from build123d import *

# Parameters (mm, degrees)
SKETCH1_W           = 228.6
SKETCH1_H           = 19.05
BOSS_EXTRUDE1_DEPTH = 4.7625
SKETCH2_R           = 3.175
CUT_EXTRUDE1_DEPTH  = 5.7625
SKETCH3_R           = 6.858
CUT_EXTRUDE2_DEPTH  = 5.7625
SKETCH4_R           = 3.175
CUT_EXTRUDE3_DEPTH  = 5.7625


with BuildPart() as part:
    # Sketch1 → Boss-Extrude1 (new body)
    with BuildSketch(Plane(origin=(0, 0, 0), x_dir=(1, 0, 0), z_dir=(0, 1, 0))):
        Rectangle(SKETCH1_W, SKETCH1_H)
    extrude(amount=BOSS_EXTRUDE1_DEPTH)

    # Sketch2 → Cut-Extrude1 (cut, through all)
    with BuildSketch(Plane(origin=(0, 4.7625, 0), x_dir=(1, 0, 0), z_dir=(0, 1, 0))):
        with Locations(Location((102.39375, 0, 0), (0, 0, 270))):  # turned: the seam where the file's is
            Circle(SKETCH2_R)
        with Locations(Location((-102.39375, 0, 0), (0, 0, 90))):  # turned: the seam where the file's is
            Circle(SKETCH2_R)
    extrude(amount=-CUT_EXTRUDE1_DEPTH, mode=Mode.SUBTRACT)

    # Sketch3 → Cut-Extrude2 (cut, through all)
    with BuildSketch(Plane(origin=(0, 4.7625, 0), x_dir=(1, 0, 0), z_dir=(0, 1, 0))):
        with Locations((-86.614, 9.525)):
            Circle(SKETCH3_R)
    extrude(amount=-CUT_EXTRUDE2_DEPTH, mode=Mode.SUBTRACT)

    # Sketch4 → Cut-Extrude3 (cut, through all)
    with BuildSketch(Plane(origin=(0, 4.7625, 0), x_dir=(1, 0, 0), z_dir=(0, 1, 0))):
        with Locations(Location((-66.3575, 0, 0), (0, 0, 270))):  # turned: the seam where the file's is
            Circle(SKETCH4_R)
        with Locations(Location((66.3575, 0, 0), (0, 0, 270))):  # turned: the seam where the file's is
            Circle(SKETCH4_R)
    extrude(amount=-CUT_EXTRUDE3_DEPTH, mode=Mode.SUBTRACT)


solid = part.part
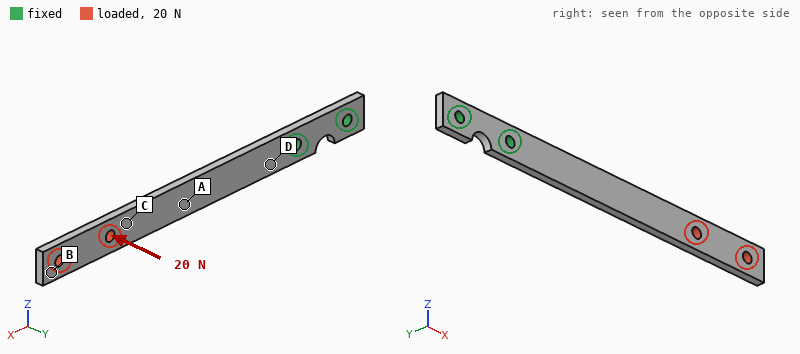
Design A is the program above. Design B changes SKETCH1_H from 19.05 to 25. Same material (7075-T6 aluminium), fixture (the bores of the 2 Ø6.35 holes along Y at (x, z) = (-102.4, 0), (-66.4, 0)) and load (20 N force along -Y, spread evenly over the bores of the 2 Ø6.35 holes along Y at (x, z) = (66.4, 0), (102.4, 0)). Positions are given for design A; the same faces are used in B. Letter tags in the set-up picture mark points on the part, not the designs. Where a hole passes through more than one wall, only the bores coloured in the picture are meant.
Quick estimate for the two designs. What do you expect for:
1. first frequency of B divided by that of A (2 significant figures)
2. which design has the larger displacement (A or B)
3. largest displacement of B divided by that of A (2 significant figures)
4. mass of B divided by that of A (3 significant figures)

0.99
A
0.77
1.32
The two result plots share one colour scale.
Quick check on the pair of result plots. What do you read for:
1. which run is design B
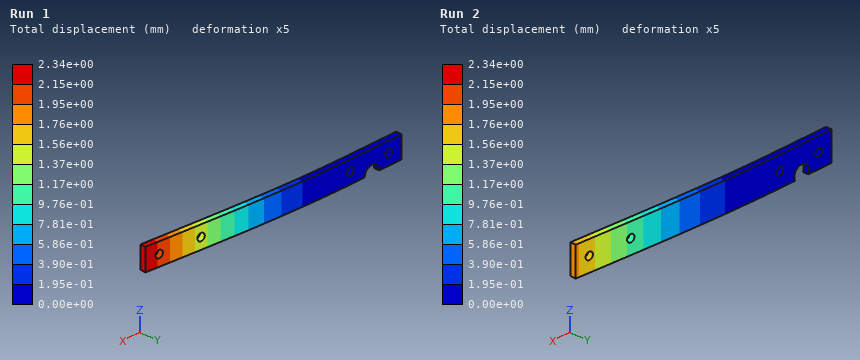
Run 2
